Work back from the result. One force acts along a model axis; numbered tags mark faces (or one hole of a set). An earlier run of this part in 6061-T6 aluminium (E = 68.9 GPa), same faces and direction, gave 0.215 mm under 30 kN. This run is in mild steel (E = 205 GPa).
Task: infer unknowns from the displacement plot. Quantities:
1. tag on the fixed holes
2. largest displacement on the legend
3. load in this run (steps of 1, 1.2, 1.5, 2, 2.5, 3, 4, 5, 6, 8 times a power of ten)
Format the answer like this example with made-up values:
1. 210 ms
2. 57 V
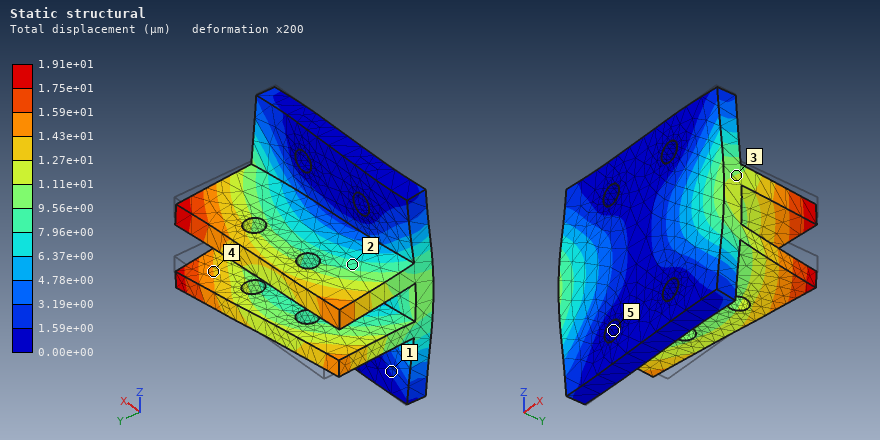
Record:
1. 5
2. 1.91e+01 µm
3. 8 kN
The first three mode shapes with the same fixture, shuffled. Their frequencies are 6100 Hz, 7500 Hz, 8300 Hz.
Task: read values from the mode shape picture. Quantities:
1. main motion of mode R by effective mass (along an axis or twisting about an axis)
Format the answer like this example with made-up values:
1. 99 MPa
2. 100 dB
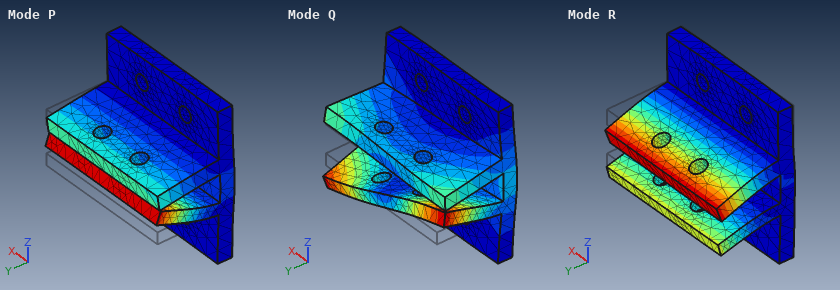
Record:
1. along Z
